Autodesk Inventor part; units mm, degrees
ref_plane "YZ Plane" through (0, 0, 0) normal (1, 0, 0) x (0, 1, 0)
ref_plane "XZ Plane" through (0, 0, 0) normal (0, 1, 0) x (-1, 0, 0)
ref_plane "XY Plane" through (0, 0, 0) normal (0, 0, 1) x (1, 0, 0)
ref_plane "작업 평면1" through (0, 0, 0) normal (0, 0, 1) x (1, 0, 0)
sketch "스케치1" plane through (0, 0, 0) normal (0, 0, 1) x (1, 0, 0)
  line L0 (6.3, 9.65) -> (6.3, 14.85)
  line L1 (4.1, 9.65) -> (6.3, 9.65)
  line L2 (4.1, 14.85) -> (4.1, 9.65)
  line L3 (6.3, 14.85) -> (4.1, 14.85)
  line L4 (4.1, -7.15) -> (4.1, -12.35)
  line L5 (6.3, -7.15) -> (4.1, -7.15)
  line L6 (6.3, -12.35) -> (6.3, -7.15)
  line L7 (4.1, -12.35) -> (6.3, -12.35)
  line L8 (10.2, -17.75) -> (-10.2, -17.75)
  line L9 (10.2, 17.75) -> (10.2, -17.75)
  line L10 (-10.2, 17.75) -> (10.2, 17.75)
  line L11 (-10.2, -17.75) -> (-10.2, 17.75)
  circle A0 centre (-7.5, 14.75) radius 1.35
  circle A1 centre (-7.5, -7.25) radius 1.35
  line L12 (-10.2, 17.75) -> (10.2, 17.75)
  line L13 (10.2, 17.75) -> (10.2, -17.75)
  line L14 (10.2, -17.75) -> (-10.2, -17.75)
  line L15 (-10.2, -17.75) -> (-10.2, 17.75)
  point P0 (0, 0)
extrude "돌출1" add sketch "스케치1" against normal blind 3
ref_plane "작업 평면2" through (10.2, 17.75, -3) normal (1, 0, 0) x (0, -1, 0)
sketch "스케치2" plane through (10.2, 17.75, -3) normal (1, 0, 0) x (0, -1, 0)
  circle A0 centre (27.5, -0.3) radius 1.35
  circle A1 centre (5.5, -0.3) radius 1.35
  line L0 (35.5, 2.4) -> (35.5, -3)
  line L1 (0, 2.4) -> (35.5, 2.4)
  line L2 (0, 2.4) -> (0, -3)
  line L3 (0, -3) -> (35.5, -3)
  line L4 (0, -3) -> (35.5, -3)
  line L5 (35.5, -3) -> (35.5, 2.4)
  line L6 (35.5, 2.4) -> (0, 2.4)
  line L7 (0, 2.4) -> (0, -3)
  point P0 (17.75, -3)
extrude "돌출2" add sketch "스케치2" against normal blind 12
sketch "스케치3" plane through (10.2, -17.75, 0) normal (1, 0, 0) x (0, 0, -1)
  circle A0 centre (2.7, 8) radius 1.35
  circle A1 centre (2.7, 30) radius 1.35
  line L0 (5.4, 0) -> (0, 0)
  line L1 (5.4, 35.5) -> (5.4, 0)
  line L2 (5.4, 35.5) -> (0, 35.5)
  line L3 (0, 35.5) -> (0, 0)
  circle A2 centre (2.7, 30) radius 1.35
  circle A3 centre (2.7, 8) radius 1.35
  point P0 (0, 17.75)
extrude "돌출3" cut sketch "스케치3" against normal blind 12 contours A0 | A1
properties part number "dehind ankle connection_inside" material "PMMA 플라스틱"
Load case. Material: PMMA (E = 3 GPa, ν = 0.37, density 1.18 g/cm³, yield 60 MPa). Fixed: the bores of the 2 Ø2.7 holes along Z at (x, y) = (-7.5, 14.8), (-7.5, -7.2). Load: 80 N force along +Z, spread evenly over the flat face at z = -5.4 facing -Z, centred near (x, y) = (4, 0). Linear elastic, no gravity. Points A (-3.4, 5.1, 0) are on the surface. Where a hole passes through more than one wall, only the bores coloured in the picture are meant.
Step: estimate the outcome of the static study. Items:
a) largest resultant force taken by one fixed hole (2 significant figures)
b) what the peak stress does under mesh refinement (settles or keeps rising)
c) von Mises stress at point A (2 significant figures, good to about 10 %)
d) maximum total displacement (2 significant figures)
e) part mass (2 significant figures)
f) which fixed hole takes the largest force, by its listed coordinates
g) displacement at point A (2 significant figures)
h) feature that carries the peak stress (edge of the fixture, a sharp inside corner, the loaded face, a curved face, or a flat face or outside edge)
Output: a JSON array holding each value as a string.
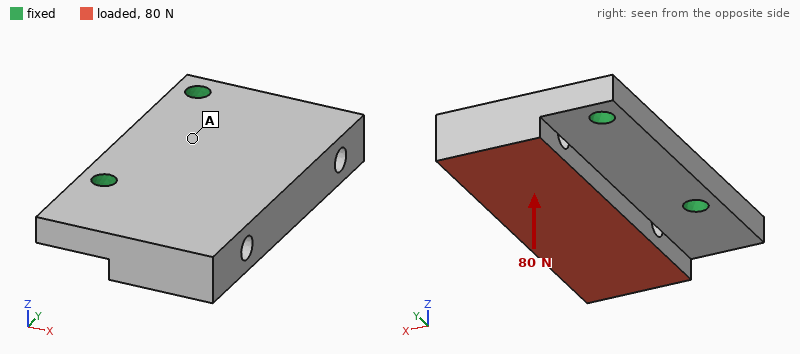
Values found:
["52 N", "keeps rising", "6.5 MPa", "0.43 mm", "3.6 g", "(-7.5, -7.2)", "0.069 mm", "edge of the fixture"]
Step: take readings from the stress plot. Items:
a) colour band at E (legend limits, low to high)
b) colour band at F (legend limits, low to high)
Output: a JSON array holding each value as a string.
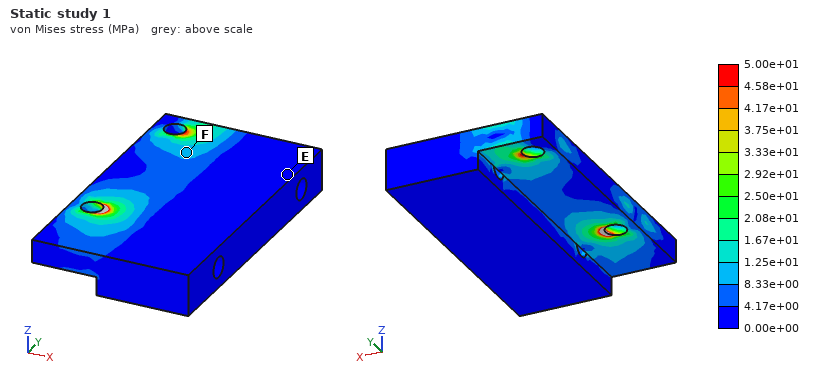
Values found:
["0.00e+00 to 4.17e+00 MPa", "8.33e+00 to 1.25e+01 MPa"]
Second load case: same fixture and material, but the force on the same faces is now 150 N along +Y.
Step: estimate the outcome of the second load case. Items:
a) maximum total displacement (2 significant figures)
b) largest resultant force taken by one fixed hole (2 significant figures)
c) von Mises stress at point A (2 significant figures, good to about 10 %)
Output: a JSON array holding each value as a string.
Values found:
["98 µm", "110 N", "1.4 MPa"]
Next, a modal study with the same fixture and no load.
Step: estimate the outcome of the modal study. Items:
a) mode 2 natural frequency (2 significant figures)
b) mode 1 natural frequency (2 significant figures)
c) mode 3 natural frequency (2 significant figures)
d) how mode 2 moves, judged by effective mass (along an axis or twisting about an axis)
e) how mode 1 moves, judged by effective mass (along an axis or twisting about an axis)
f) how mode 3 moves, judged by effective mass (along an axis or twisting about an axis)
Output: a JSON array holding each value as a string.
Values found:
["3500 Hz", "1600 Hz", "6900 Hz", "twisting about X", "along Z", "along Y"]
